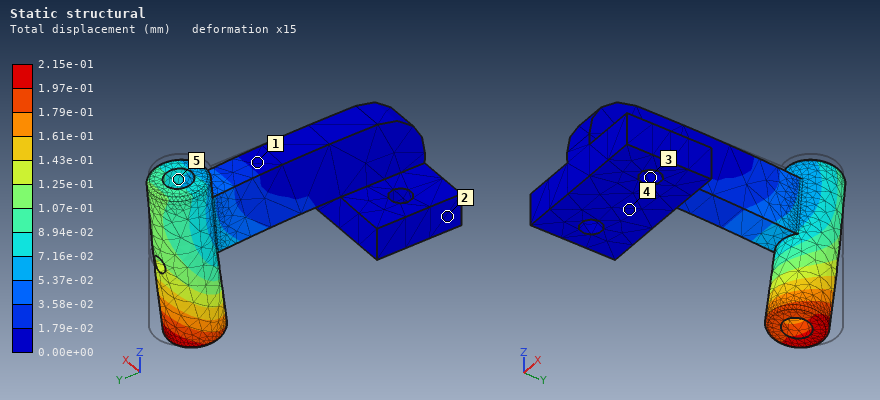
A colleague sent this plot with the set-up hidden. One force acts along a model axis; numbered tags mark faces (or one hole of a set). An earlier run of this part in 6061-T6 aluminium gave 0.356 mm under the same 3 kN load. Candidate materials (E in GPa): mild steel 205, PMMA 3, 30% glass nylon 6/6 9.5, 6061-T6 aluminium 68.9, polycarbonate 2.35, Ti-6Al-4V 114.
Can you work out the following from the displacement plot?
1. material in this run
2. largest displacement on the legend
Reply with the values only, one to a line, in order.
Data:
Ti-6Al-4V
2.15e-01 mm
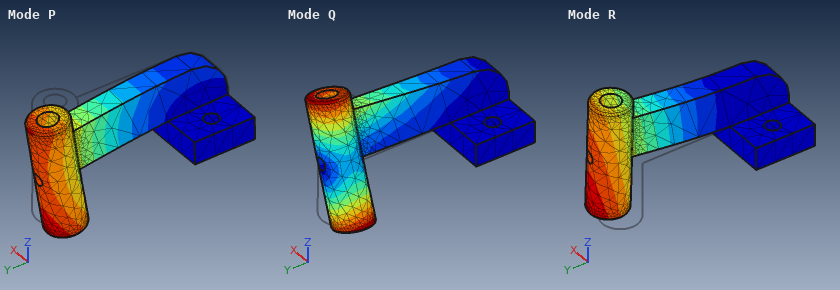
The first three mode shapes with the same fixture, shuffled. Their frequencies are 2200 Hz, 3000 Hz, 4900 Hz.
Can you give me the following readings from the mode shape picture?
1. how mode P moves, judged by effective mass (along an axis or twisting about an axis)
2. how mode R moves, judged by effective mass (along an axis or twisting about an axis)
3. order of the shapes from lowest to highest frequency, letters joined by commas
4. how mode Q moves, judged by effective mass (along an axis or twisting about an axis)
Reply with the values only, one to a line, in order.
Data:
along Z
along X
R, P, Q
twisting about Y
